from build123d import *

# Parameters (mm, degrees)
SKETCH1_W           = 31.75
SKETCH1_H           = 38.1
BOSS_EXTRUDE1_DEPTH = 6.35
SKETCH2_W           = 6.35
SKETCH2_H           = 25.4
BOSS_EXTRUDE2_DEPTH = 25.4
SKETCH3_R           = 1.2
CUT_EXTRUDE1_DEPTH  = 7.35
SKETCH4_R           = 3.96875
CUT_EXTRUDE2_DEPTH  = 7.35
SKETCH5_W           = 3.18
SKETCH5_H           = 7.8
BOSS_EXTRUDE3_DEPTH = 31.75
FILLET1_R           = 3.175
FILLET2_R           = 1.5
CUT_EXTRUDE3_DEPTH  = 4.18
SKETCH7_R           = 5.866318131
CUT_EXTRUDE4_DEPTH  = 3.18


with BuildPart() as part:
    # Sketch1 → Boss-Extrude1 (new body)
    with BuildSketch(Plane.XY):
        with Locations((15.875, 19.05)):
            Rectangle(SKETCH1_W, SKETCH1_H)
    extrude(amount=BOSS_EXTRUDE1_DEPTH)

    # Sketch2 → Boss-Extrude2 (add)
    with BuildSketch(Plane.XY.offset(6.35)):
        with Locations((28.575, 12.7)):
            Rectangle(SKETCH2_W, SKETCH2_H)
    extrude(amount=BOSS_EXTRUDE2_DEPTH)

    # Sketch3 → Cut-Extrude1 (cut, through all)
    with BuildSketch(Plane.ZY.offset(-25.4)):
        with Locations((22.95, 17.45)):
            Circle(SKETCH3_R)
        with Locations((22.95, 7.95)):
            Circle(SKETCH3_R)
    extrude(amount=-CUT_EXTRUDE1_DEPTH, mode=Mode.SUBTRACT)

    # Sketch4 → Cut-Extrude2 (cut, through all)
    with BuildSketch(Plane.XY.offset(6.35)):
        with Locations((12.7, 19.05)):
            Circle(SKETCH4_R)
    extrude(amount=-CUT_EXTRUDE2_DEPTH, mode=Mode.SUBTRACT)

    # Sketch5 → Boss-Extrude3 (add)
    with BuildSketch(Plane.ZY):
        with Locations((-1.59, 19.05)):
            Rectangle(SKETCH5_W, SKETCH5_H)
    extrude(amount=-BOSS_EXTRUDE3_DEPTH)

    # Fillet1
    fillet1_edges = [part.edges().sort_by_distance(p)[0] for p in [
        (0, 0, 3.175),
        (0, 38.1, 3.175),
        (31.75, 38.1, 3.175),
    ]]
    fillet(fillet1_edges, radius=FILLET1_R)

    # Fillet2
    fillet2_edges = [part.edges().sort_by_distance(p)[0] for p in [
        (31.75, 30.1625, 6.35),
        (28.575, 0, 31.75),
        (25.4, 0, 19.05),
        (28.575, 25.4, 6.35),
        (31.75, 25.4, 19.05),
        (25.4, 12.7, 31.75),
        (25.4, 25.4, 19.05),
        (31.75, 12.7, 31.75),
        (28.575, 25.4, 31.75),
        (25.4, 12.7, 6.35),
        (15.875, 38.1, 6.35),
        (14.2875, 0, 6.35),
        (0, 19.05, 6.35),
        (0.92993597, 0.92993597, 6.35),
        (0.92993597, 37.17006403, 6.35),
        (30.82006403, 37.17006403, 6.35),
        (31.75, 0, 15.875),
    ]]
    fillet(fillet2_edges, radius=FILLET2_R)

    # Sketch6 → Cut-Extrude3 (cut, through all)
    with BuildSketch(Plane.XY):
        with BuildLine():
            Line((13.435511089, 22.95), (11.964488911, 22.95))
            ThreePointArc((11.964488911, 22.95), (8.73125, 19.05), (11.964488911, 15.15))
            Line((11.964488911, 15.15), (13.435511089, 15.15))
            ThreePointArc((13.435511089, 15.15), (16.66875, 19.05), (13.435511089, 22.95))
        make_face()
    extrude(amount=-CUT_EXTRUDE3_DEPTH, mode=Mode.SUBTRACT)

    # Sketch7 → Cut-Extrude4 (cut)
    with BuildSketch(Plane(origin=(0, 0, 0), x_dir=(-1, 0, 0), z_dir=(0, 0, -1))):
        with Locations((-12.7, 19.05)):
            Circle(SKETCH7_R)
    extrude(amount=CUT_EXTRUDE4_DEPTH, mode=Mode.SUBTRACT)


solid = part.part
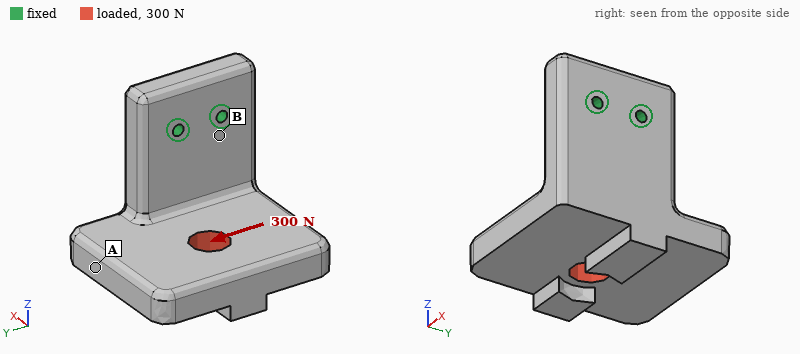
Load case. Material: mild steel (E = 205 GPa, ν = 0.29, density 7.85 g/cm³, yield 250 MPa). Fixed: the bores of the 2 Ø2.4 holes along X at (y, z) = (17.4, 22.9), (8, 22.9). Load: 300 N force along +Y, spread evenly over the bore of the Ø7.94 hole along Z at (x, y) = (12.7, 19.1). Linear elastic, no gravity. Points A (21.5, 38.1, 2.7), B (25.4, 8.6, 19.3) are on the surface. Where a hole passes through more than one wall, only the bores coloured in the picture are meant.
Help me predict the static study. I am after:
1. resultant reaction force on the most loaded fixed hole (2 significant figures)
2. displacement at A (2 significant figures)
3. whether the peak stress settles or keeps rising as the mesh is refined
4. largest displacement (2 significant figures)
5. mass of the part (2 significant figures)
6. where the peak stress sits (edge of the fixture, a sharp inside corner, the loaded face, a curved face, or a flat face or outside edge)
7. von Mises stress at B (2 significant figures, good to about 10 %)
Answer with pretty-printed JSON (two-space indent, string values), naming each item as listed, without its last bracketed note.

{
  "resultant reaction force on the most loaded fixed hole": "620 N",
  "displacement at A": "12 µm",
  "whether the peak stress settles or keeps rising as the mesh is refined": "keeps rising",
  "largest displacement": "18 µm",
  "mass of the part": "92 g",
  "where the peak stress sits": "edge of the fixture",
  "von Mises stress at B": "23 MPa"
}
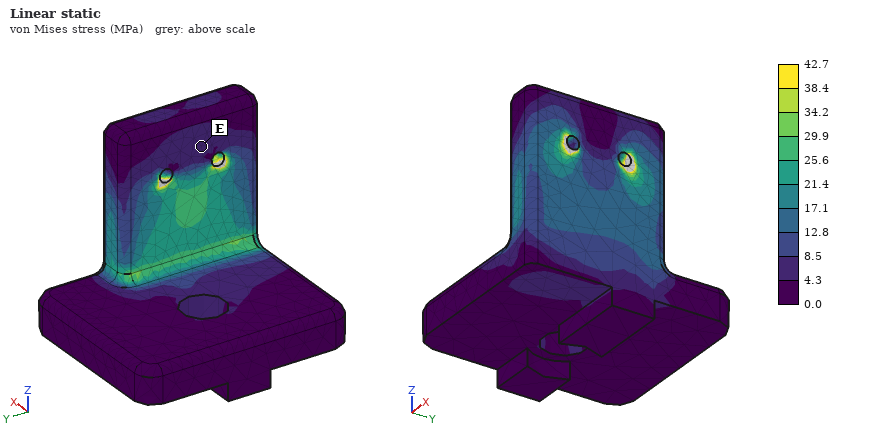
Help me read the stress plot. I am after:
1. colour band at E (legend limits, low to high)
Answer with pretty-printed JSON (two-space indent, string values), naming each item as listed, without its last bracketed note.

{
  "colour band at E": "4.3 to 8.5 MPa"
}
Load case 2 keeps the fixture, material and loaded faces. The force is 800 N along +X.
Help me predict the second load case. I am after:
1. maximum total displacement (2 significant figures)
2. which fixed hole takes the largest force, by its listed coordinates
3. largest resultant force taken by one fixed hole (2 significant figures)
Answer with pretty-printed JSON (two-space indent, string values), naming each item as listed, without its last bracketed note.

{
  "maximum total displacement": "62 µm",
  "which fixed hole takes the largest force, by its listed coordinates": "(17.4, 22.9)",
  "largest resultant force taken by one fixed hole": "710 N"
}
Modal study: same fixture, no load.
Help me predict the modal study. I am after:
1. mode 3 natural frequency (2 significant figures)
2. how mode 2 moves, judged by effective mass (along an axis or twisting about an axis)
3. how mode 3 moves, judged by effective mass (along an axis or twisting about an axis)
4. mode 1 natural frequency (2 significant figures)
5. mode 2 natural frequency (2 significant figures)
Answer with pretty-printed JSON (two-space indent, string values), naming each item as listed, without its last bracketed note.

{
  "mode 3 natural frequency": "6900 Hz",
  "how mode 2 moves, judged by effective mass": "along Y",
  "how mode 3 moves, judged by effective mass": "along X",
  "mode 1 natural frequency": "2300 Hz",
  "mode 2 natural frequency": "3300 Hz"
}
